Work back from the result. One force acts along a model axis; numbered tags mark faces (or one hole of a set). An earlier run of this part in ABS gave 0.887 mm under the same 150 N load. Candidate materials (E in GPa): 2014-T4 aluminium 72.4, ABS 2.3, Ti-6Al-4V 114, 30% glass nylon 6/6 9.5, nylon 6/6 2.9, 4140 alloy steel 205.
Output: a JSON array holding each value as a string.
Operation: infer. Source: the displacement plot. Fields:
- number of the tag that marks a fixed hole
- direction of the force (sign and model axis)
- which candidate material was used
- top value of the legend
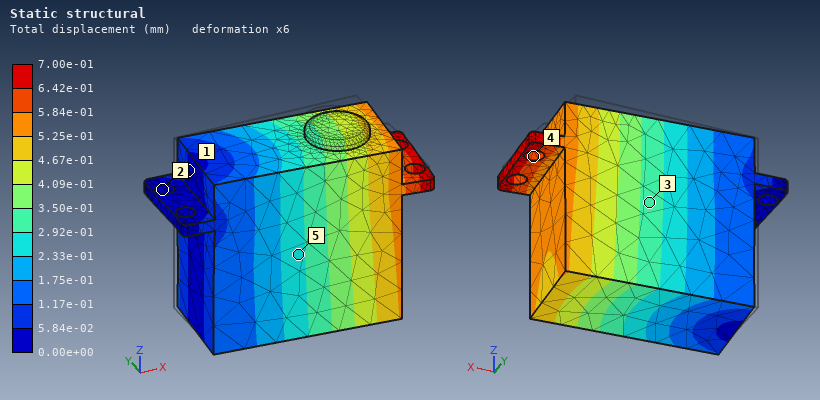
["2", "-Y", "nylon 6/6", "7.00e-01 mm"]
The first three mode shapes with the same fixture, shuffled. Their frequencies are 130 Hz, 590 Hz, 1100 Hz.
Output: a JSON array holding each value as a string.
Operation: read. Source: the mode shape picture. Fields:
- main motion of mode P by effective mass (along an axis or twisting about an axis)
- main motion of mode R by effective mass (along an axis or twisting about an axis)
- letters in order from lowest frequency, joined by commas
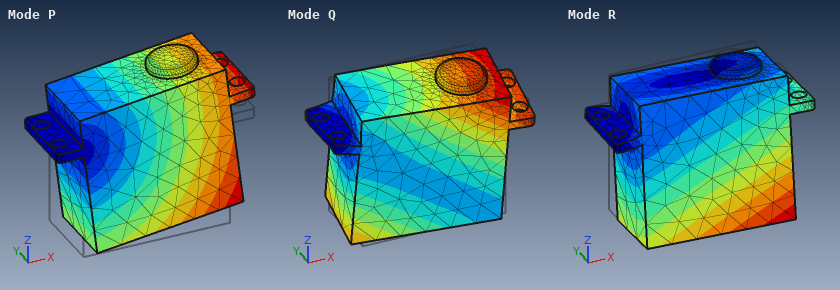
["along Z", "along Y", "P, R, Q"]
